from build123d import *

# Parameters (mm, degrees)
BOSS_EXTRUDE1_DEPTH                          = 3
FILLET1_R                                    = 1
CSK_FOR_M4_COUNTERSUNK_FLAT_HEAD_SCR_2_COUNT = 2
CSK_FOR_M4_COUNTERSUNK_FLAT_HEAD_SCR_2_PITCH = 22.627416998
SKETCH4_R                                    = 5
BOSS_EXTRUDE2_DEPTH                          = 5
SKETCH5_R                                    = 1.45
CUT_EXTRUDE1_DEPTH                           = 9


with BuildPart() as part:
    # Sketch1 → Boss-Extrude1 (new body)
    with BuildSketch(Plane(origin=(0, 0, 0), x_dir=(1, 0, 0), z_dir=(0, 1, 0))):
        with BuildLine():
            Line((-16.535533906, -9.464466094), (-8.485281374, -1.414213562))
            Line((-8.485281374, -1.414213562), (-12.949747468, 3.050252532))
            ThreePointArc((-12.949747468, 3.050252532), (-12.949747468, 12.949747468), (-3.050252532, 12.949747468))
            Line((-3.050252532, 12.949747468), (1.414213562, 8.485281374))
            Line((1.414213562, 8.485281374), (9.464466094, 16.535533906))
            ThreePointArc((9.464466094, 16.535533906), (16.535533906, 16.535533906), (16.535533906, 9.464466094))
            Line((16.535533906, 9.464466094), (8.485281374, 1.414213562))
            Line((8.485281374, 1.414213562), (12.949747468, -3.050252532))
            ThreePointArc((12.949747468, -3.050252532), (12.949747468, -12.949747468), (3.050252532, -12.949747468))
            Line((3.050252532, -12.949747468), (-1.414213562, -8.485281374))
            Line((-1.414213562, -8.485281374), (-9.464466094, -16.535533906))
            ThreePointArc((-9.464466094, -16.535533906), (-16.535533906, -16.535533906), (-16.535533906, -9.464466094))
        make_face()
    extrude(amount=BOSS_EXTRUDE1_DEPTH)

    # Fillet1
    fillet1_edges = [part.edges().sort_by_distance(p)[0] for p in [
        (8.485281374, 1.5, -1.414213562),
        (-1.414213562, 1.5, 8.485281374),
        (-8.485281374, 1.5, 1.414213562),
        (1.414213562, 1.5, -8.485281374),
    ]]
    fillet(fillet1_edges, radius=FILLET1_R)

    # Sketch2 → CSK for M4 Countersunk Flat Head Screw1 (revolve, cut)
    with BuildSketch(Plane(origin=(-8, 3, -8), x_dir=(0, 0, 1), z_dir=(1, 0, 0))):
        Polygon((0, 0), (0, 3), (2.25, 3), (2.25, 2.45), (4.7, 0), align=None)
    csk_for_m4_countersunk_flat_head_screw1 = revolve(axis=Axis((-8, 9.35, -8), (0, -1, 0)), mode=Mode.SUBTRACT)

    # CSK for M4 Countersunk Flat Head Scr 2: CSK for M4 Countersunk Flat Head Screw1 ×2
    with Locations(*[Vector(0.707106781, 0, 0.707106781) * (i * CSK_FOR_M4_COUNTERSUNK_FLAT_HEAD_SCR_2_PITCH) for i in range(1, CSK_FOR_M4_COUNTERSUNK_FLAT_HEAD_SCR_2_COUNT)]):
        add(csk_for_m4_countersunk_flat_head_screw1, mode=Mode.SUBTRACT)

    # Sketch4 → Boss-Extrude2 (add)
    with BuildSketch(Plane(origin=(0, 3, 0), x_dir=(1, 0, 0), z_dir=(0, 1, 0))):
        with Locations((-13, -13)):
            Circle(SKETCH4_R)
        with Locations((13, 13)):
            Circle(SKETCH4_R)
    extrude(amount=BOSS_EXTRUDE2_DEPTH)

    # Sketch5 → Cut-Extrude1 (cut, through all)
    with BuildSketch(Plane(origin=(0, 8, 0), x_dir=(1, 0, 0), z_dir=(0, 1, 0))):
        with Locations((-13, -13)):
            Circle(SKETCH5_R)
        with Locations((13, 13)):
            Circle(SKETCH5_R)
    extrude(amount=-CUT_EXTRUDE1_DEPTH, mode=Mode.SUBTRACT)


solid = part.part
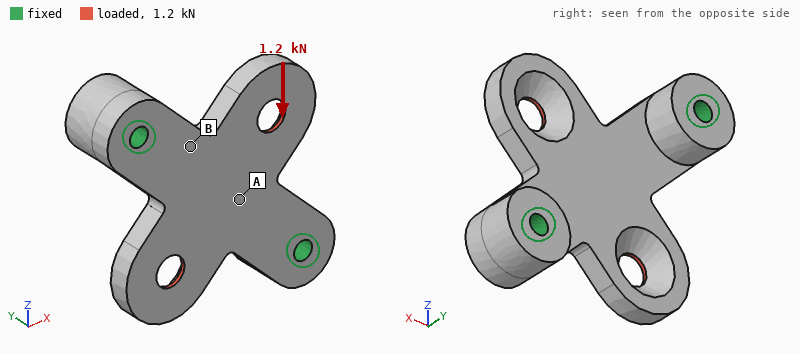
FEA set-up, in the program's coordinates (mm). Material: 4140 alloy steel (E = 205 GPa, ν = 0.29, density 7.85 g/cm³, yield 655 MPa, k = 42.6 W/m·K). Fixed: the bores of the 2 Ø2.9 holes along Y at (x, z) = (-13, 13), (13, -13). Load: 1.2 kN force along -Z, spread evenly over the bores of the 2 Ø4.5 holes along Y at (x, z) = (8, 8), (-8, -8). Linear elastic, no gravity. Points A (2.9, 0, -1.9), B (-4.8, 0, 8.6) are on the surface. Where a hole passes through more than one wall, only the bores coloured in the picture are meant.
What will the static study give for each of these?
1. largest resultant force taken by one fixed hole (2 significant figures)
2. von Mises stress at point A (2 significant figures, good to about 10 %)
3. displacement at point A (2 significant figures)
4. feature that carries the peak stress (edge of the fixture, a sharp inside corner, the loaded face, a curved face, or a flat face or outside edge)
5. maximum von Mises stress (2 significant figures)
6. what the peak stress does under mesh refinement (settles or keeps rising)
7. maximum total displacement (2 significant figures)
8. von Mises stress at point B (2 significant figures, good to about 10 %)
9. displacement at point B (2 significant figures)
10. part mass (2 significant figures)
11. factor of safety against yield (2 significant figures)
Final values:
600 N
19 MPa
5.9 µm
a curved face
220 MPa
settles
26 µm
57 MPa
4.4 µm
22 g
2.9
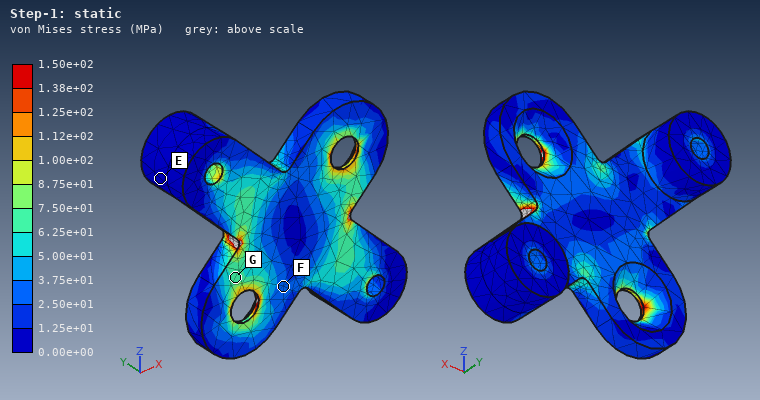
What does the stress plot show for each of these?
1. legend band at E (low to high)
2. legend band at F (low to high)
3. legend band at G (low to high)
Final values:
0.00e+00 to 1.25e+01 MPa
2.50e+01 to 3.75e+01 MPa
6.25e+01 to 7.50e+01 MPa
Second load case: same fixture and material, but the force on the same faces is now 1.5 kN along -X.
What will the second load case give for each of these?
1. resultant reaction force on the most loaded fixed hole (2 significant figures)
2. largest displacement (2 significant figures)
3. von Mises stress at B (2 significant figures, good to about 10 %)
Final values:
750 N
32 µm
87 MPa
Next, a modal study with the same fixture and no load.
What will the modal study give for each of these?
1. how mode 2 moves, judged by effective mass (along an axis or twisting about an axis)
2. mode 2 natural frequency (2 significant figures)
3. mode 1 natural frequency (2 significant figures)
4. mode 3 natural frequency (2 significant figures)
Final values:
along Y
7800 Hz
5700 Hz
18 kHz
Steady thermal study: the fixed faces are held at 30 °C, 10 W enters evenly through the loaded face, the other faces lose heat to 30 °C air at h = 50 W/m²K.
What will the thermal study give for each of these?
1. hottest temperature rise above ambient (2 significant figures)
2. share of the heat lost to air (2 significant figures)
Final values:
69 K
29 %
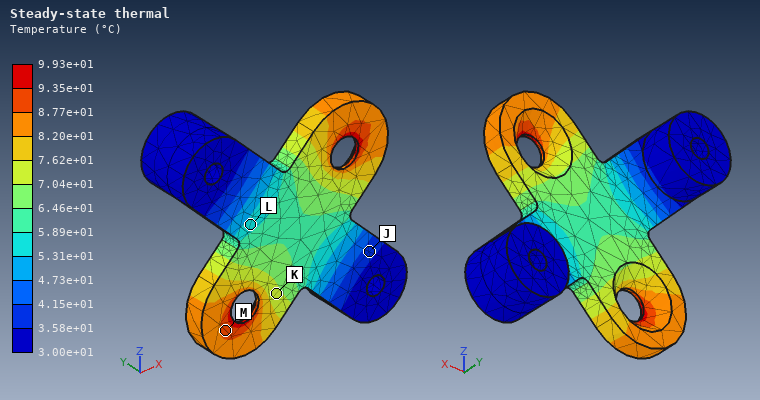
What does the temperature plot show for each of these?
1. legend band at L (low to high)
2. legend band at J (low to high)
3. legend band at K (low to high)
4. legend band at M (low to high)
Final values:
5.31e+01 to 5.89e+01 °C
3.58e+01 to 4.15e+01 °C
7.04e+01 to 7.62e+01 °C
8.77e+01 to 9.35e+01 °C
